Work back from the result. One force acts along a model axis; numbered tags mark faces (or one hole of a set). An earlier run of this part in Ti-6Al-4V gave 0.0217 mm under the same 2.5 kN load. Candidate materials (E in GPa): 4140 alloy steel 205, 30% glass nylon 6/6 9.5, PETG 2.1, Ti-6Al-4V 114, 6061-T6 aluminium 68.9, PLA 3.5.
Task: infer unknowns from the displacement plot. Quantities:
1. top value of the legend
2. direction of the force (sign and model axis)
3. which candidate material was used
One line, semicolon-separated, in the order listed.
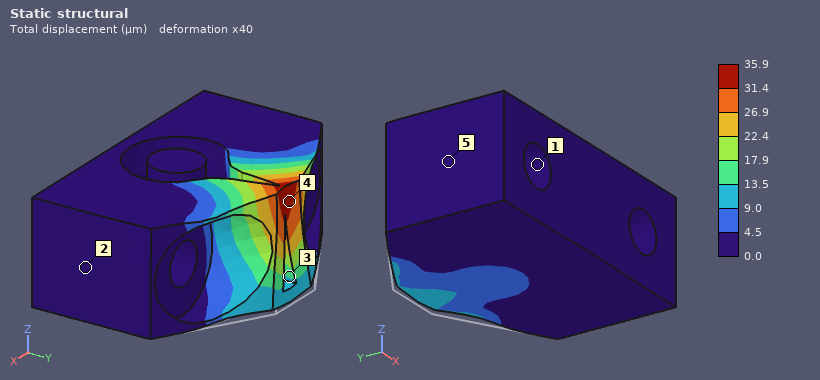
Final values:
35.9 µm; -Y; 6061-T6 aluminium
